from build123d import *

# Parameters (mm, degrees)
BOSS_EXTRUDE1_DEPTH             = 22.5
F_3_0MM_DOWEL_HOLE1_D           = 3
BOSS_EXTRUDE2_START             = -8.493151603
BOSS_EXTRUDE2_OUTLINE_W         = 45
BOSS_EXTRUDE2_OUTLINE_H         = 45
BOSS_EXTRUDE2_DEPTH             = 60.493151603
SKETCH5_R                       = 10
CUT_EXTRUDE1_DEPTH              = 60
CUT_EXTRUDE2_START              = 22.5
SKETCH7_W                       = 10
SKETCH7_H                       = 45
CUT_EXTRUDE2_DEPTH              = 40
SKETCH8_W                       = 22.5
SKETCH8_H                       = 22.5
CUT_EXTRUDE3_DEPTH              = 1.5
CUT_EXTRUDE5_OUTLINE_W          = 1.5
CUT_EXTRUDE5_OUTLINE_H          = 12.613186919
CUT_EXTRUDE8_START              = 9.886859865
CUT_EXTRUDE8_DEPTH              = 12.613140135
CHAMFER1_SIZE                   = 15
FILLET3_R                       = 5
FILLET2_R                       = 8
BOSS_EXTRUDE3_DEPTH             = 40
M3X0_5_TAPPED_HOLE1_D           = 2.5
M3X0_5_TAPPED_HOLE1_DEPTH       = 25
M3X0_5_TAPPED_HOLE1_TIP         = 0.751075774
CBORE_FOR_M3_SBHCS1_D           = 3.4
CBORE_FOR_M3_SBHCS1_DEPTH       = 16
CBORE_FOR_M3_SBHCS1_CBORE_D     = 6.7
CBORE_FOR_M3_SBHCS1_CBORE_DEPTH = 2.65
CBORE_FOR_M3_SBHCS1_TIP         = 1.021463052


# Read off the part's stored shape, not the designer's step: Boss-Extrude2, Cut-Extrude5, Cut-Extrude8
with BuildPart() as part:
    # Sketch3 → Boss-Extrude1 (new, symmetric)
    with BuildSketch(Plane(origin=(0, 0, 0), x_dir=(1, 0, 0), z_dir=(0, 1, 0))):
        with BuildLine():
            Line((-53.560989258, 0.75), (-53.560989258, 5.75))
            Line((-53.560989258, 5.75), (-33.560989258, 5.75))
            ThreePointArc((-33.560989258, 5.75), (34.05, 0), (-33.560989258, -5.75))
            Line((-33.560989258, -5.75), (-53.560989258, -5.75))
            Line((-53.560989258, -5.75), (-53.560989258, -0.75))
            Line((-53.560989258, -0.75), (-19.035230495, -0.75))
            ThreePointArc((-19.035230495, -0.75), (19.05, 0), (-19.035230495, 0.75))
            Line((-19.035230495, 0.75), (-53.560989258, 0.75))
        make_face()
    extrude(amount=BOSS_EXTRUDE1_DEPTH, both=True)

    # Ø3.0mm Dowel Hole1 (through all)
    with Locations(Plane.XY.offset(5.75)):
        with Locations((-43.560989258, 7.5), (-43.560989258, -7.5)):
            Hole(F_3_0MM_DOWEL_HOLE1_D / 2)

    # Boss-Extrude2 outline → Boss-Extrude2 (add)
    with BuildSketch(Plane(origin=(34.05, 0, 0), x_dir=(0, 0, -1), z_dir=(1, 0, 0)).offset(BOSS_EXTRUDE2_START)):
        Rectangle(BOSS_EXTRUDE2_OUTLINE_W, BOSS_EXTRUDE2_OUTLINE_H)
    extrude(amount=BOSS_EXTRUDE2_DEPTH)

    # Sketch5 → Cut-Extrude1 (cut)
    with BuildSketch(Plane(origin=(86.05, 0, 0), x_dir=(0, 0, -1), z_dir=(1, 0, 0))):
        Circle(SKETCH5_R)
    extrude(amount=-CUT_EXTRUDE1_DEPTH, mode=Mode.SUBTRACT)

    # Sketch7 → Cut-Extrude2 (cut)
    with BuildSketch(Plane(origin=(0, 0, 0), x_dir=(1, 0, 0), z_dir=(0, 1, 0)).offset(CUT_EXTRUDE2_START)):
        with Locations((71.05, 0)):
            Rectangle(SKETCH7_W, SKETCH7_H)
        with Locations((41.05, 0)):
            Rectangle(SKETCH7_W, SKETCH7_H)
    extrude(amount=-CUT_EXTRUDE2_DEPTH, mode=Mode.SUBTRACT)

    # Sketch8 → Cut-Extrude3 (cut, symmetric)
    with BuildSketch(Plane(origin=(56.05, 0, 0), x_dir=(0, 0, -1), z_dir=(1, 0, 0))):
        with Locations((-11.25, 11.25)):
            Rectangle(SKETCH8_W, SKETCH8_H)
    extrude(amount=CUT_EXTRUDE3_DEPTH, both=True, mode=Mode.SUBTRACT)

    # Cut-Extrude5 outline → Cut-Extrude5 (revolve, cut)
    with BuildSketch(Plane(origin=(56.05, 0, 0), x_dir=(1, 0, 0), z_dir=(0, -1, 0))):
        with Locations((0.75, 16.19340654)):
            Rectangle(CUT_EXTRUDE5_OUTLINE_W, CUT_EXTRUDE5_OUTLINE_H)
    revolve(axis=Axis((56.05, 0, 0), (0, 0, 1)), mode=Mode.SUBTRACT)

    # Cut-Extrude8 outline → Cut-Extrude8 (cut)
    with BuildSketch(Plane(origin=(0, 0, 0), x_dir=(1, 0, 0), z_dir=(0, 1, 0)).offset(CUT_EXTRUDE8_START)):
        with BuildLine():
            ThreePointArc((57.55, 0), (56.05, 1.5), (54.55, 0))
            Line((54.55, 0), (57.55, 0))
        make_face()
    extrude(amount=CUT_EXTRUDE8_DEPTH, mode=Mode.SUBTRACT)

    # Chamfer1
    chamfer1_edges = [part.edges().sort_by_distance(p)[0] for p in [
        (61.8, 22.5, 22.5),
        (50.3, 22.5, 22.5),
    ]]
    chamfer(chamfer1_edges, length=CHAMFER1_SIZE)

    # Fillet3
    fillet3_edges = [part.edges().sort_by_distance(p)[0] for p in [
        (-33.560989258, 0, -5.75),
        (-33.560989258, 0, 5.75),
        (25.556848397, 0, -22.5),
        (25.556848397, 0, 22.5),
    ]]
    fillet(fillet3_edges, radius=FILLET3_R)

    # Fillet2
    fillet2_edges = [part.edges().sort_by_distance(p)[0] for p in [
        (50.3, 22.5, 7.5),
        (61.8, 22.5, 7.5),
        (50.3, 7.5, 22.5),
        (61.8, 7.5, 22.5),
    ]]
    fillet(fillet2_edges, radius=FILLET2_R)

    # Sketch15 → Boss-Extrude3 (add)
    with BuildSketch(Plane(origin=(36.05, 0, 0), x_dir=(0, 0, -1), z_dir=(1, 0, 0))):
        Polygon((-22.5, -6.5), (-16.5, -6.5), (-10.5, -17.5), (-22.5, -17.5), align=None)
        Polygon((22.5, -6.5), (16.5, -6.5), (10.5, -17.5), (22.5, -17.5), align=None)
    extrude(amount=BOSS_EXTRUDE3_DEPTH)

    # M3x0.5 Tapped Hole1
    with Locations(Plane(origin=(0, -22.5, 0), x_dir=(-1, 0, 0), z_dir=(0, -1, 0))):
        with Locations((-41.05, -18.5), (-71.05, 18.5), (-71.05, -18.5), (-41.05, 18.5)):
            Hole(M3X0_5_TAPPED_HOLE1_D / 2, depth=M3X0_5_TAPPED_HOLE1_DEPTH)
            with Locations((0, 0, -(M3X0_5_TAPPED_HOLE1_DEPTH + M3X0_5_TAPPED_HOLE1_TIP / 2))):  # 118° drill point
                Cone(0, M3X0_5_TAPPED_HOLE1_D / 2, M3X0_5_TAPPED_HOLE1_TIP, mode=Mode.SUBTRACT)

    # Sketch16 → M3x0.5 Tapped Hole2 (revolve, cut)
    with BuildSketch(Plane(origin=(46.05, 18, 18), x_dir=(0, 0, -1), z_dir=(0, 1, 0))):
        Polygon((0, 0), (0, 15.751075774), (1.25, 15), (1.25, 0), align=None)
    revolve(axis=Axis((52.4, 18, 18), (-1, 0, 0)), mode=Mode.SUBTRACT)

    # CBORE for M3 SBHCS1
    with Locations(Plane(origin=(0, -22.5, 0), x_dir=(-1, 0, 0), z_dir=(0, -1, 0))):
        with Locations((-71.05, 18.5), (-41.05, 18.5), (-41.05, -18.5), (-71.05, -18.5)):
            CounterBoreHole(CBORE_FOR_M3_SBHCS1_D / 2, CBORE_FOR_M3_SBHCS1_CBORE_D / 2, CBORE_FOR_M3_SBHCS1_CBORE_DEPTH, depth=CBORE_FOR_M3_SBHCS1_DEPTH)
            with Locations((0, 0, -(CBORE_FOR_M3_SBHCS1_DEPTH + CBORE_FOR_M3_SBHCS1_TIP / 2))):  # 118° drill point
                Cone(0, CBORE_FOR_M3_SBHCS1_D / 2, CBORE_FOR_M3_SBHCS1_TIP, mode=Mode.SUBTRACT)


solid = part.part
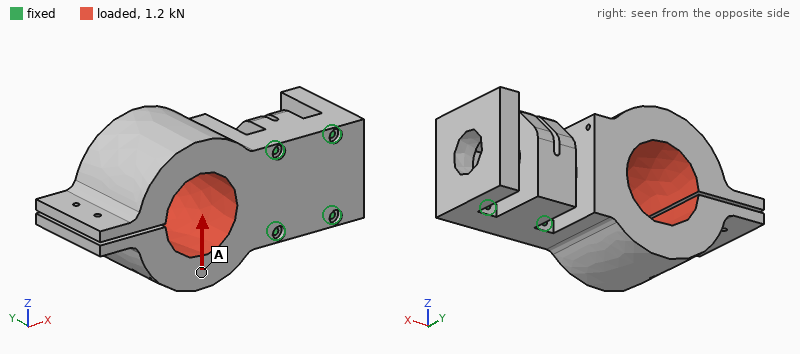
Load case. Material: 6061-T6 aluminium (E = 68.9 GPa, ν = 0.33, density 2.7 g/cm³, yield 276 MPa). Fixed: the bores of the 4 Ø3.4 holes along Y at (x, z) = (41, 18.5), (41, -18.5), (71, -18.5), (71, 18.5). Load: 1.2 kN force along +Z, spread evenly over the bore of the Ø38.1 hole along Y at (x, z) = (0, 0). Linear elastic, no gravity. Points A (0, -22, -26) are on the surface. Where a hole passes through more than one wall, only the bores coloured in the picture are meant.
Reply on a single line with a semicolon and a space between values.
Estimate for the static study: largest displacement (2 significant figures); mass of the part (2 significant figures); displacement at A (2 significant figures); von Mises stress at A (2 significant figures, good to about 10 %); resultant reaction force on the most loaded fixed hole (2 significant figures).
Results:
40 µm; 490 g; 11 µm; 1.6 MPa; 1.4 kN
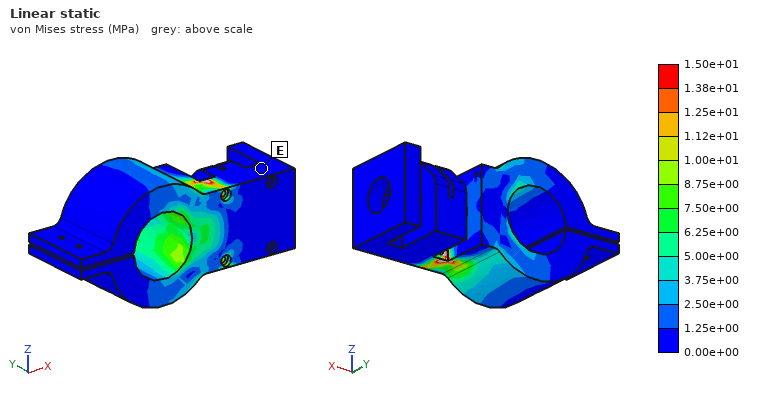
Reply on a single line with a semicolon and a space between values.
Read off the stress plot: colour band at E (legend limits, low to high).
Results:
0.00e+00 to 1.25e+00 MPa
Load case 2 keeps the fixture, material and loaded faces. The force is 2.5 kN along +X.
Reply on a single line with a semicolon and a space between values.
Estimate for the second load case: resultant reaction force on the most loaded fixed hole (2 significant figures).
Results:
1.5 kN
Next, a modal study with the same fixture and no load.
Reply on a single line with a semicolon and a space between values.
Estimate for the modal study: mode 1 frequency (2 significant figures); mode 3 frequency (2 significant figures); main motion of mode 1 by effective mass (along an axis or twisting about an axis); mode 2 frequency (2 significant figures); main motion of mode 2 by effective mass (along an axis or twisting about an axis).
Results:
1000 Hz; 2000 Hz; along Y; 1700 Hz; along Z
